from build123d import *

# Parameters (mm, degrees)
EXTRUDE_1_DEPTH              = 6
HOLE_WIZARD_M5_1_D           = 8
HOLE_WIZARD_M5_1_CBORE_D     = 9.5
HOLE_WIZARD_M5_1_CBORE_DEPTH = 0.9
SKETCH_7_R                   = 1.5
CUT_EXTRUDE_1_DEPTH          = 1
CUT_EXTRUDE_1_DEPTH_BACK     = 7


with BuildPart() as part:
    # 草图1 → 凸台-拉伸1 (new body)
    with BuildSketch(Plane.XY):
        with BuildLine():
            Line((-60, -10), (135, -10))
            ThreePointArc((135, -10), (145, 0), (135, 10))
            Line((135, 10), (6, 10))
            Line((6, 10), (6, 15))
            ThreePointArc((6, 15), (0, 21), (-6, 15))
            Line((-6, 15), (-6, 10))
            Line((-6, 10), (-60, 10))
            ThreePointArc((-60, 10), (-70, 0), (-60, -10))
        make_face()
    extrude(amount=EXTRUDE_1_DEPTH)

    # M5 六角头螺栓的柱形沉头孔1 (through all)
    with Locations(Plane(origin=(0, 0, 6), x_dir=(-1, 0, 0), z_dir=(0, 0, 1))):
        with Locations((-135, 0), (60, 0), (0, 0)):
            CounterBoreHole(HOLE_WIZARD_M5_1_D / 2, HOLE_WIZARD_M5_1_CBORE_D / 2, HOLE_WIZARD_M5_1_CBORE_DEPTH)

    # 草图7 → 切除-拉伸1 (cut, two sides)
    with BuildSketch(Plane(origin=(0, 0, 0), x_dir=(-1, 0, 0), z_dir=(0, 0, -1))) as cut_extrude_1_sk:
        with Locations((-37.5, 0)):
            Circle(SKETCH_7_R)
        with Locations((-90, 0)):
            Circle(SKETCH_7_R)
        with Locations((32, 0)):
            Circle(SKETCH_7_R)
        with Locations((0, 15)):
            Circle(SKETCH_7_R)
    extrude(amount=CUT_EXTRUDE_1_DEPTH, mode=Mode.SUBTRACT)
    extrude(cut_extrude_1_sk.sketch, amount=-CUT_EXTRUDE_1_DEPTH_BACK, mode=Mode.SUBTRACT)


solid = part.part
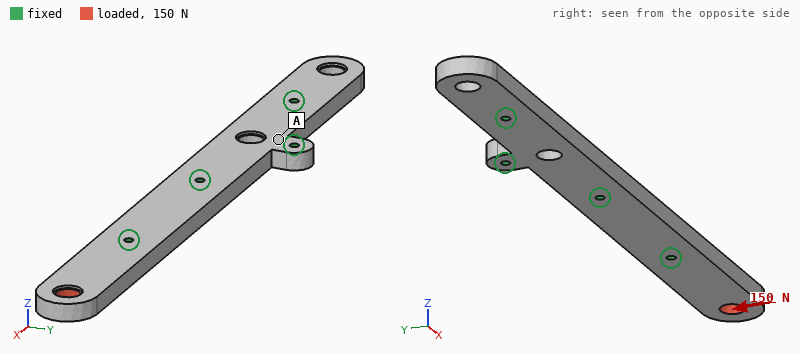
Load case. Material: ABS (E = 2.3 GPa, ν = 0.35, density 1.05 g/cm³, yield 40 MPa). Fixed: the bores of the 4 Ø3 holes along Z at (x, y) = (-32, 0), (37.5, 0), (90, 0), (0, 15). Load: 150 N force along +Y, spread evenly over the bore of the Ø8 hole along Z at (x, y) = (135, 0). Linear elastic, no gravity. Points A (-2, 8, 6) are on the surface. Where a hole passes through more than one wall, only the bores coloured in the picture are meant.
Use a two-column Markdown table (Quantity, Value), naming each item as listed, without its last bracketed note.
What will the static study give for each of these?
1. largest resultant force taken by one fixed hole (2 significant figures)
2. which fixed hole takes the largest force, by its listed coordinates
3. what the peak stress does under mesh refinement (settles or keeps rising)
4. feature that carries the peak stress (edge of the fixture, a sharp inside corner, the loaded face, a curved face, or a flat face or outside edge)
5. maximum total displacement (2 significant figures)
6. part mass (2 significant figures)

| Quantity | Value |
|---|---|
| largest resultant force taken by one fixed hole | 270 N |
| which fixed hole takes the largest force, by its listed coordinates | (90, 0) |
| what the peak stress does under mesh refinement | keeps rising |
| feature that carries the peak stress | edge of the fixture |
| maximum total displacement | 1.3 mm |
| part mass | 26 g |
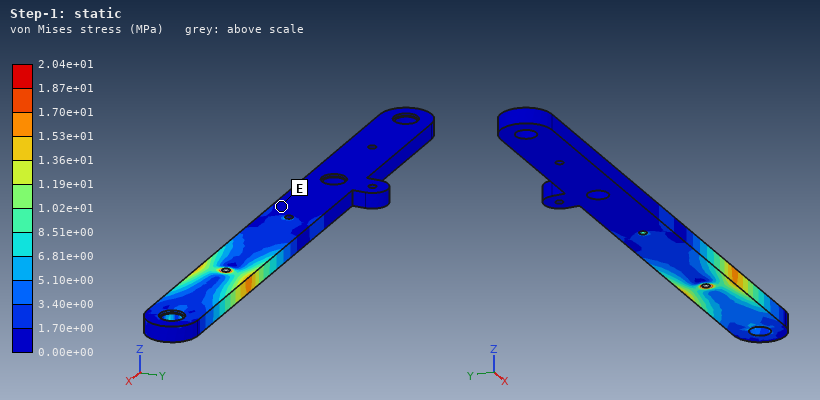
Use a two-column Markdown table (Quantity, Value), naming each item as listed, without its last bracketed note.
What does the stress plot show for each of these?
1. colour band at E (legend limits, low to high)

| Quantity | Value |
|---|---|
| colour band at E | 0.00e+00 to 1.70e+00 MPa |
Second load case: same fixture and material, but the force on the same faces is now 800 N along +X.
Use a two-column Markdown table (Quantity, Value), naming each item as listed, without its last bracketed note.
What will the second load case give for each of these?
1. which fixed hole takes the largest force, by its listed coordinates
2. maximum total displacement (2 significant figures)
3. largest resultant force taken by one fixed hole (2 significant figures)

| Quantity | Value |
|---|---|
| which fixed hole takes the largest force, by its listed coordinates | (90, 0) |
| maximum total displacement | 0.72 mm |
| largest resultant force taken by one fixed hole | 720 N |
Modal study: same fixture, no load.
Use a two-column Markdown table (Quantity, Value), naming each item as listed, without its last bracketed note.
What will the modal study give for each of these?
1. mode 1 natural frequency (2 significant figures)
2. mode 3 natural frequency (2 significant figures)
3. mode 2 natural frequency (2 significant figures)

| Quantity | Value |
|---|---|
| mode 1 natural frequency | 520 Hz |
| mode 3 natural frequency | 1200 Hz |
| mode 2 natural frequency | 1100 Hz |
